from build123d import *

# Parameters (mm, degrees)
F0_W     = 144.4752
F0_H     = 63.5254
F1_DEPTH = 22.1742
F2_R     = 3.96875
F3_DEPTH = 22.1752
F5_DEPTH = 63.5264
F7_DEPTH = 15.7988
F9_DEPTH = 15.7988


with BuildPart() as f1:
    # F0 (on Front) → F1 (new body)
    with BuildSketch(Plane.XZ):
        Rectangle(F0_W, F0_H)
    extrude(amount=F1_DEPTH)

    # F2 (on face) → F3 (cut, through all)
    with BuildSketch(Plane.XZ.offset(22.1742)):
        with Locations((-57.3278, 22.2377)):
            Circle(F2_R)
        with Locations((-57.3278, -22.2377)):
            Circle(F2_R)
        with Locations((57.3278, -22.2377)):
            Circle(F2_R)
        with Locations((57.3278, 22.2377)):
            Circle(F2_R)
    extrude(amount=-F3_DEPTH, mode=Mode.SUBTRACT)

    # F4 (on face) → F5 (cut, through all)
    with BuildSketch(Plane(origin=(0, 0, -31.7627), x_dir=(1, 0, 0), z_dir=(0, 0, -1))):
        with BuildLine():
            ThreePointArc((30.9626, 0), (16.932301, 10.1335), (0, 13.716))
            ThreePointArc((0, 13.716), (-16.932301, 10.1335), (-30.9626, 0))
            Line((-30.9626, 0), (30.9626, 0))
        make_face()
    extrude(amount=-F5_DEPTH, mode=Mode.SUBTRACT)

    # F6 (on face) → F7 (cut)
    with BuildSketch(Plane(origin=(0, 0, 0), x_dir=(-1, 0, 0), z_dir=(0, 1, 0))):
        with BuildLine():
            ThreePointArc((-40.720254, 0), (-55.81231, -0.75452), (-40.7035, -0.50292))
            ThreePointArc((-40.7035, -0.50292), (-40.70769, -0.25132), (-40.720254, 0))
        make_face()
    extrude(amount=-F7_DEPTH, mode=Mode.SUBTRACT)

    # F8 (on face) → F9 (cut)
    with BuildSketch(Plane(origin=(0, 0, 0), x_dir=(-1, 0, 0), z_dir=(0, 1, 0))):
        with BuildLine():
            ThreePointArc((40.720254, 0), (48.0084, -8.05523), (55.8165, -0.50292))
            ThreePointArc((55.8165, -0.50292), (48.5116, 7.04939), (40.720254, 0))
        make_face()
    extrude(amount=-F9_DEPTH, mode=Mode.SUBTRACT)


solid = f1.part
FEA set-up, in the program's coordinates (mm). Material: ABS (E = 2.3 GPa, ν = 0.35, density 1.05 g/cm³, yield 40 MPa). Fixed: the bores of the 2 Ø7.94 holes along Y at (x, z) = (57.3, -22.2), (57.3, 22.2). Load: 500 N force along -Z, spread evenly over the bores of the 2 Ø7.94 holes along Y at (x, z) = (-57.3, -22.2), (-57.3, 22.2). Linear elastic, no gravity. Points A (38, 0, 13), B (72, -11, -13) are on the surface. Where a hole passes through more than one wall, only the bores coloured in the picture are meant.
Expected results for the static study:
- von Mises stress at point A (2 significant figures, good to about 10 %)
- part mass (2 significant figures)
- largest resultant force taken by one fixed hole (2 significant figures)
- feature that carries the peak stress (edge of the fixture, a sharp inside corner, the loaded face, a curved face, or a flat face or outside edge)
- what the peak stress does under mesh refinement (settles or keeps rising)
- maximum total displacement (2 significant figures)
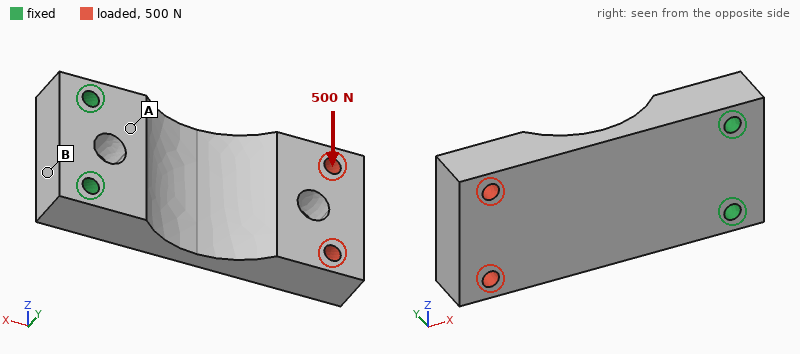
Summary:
1.7 MPa
160 g
1.2 kN
edge of the fixture
keeps rising
0.72 mm
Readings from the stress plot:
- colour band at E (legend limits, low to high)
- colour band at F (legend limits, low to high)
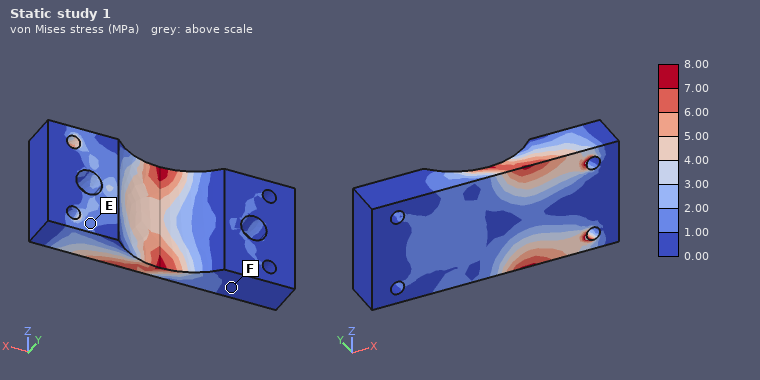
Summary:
1.00 to 2.00 MPa
0.00 to 1.00 MPa
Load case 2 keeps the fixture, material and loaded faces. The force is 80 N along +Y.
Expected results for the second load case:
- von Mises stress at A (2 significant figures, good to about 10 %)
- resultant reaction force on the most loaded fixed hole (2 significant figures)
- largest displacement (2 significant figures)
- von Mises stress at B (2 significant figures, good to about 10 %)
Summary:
1.6 MPa
41 N
1.6 mm
0.48 MPa
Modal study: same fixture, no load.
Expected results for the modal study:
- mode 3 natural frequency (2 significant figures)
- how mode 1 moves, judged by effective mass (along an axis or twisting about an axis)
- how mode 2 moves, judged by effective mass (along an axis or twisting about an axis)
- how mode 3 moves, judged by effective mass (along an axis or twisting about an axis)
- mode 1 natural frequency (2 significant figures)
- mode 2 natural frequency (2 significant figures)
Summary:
790 Hz
along Y
along Z
along Z
170 Hz
570 Hz
